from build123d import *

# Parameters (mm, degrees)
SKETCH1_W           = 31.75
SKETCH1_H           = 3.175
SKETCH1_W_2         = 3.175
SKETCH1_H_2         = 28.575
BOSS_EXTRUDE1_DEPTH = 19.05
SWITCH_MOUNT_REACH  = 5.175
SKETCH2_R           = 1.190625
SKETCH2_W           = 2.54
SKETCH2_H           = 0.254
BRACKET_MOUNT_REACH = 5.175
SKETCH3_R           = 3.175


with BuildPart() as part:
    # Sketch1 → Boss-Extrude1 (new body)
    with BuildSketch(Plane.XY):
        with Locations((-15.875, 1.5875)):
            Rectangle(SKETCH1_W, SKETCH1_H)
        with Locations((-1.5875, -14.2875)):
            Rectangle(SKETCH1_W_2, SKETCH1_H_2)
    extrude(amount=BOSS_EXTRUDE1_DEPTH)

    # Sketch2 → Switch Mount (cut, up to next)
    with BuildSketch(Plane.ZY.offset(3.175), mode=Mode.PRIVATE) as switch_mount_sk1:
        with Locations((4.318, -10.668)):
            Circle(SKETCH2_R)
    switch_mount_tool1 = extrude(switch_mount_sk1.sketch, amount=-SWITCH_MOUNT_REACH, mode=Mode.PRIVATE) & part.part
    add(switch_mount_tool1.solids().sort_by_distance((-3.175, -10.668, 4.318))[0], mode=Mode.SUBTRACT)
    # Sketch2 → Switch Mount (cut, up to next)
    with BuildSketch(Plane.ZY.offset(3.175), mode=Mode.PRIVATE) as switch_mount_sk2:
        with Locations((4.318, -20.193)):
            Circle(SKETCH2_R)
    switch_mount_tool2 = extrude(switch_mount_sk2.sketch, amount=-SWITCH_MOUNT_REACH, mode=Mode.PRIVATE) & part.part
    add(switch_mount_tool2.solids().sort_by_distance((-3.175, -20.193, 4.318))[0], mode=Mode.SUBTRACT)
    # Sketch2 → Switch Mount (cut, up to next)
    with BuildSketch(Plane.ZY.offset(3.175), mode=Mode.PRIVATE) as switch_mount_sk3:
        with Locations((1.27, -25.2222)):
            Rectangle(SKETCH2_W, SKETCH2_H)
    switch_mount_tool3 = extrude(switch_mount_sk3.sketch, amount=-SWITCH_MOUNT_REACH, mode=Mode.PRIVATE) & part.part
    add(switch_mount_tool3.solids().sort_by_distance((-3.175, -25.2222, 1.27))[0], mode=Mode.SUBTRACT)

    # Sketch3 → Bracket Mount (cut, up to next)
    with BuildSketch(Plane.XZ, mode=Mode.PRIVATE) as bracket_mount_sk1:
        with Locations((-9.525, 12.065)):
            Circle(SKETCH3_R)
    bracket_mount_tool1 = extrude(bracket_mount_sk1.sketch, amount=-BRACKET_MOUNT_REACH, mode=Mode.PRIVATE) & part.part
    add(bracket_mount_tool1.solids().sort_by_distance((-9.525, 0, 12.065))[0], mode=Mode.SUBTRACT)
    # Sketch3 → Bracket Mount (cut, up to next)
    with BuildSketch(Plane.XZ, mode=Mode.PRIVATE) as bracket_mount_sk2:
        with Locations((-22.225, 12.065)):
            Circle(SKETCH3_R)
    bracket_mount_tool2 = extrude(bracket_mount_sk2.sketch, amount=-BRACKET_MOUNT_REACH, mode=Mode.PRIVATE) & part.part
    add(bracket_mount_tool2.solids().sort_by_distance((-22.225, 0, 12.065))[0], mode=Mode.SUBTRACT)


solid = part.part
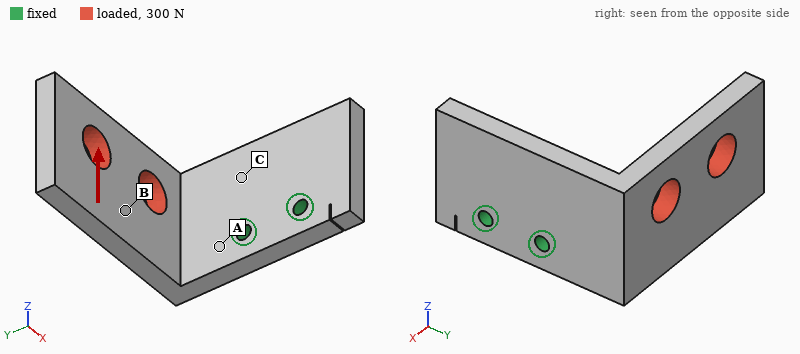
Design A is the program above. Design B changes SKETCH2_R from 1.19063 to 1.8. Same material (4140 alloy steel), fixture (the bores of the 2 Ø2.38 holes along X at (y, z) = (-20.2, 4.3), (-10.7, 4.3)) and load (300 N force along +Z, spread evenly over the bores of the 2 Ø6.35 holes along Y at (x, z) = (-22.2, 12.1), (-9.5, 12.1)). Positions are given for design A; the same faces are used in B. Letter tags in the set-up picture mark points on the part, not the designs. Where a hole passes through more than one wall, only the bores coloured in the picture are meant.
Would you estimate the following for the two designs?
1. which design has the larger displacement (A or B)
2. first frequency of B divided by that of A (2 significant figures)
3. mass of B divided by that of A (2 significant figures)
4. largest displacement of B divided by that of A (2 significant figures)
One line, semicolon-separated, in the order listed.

A; 1.0; 0.99; 0.88
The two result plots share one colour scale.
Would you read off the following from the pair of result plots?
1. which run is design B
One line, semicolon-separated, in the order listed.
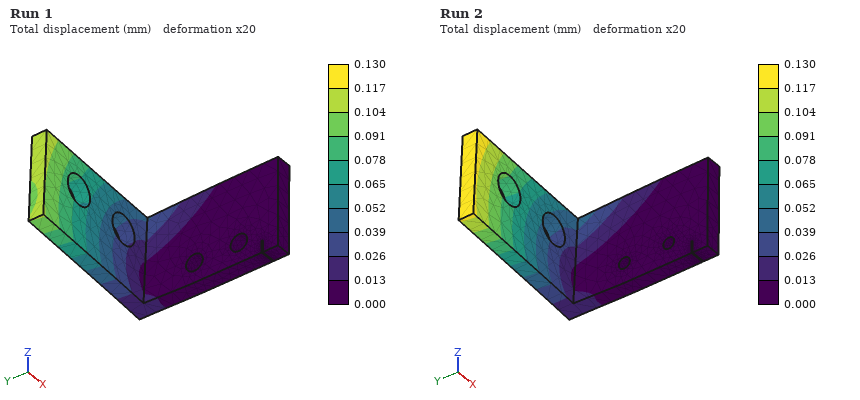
Run 1
